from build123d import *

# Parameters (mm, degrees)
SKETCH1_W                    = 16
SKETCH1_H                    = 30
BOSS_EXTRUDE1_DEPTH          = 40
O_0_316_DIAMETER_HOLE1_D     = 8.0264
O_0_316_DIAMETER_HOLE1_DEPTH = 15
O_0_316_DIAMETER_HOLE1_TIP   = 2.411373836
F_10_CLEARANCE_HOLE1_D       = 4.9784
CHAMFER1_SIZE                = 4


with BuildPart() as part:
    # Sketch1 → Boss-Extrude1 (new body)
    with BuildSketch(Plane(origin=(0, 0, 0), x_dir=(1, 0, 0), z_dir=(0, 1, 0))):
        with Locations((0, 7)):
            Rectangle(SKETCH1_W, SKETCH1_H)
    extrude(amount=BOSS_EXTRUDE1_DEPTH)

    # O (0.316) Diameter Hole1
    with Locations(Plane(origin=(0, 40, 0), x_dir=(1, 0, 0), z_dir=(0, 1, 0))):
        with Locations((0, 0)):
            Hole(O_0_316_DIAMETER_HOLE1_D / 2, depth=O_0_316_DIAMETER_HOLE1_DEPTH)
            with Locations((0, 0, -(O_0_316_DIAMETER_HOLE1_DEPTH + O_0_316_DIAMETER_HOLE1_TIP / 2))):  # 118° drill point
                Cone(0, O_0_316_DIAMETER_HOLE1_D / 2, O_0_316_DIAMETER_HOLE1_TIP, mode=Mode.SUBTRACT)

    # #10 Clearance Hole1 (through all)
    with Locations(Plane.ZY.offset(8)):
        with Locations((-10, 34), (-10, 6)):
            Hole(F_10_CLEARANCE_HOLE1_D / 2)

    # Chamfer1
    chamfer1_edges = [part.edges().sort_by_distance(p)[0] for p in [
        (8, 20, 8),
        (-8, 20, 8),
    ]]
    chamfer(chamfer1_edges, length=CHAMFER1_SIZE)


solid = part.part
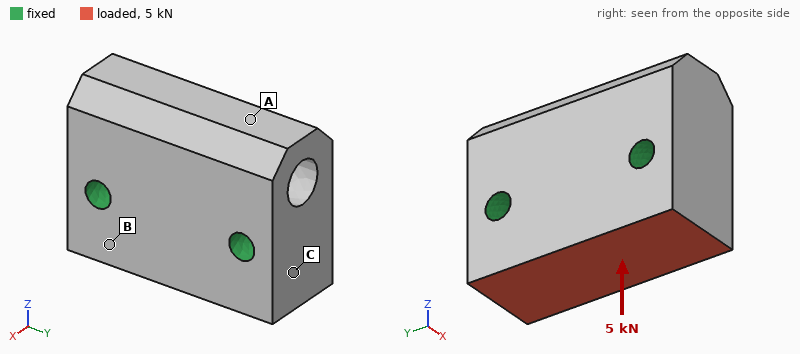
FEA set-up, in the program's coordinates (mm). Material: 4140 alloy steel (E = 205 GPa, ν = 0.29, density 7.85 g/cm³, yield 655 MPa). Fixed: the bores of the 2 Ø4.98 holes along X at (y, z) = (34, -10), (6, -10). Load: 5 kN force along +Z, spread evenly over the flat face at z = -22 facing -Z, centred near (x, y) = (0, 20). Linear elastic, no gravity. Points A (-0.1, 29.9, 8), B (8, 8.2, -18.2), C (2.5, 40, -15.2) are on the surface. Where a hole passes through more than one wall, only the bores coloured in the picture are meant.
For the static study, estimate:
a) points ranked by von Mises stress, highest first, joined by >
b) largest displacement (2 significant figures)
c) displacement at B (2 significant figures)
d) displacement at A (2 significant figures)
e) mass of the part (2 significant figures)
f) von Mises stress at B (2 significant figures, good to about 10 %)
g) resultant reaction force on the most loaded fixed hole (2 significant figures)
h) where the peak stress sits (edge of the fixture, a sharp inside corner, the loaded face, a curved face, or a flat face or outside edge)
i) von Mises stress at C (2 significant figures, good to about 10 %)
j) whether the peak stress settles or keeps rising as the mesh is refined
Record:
B > C > A
0.85 µm
0.40 µm
0.24 µm
130 g
9.1 MPa
2.5 kN
edge of the fixture
4.8 MPa
keeps rising
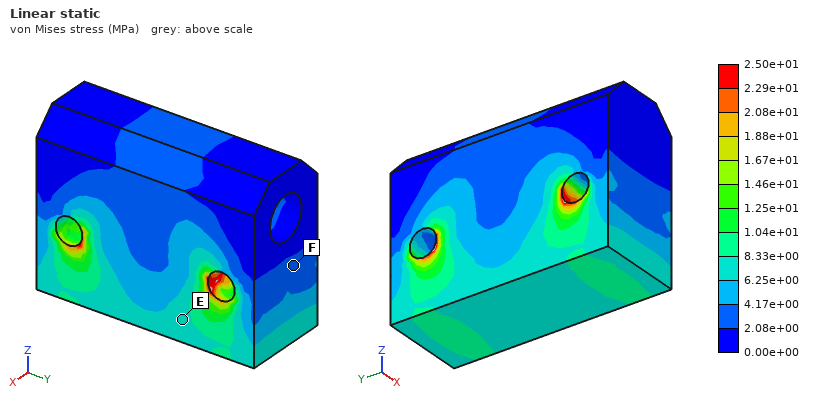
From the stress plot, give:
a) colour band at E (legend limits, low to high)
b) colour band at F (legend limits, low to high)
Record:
6.25e+00 to 8.33e+00 MPa
2.08e+00 to 4.17e+00 MPa
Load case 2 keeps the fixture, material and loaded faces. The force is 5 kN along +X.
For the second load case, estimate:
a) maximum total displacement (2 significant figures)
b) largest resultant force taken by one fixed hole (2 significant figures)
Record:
4.2 µm
2.5 kN
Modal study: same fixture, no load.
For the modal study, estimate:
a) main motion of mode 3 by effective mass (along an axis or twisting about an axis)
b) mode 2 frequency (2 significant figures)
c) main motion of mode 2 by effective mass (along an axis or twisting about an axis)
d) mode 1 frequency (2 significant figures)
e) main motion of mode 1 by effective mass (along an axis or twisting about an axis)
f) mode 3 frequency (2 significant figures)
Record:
along Y
36 kHz
twisting about Z
25 kHz
along X
38 kHz
